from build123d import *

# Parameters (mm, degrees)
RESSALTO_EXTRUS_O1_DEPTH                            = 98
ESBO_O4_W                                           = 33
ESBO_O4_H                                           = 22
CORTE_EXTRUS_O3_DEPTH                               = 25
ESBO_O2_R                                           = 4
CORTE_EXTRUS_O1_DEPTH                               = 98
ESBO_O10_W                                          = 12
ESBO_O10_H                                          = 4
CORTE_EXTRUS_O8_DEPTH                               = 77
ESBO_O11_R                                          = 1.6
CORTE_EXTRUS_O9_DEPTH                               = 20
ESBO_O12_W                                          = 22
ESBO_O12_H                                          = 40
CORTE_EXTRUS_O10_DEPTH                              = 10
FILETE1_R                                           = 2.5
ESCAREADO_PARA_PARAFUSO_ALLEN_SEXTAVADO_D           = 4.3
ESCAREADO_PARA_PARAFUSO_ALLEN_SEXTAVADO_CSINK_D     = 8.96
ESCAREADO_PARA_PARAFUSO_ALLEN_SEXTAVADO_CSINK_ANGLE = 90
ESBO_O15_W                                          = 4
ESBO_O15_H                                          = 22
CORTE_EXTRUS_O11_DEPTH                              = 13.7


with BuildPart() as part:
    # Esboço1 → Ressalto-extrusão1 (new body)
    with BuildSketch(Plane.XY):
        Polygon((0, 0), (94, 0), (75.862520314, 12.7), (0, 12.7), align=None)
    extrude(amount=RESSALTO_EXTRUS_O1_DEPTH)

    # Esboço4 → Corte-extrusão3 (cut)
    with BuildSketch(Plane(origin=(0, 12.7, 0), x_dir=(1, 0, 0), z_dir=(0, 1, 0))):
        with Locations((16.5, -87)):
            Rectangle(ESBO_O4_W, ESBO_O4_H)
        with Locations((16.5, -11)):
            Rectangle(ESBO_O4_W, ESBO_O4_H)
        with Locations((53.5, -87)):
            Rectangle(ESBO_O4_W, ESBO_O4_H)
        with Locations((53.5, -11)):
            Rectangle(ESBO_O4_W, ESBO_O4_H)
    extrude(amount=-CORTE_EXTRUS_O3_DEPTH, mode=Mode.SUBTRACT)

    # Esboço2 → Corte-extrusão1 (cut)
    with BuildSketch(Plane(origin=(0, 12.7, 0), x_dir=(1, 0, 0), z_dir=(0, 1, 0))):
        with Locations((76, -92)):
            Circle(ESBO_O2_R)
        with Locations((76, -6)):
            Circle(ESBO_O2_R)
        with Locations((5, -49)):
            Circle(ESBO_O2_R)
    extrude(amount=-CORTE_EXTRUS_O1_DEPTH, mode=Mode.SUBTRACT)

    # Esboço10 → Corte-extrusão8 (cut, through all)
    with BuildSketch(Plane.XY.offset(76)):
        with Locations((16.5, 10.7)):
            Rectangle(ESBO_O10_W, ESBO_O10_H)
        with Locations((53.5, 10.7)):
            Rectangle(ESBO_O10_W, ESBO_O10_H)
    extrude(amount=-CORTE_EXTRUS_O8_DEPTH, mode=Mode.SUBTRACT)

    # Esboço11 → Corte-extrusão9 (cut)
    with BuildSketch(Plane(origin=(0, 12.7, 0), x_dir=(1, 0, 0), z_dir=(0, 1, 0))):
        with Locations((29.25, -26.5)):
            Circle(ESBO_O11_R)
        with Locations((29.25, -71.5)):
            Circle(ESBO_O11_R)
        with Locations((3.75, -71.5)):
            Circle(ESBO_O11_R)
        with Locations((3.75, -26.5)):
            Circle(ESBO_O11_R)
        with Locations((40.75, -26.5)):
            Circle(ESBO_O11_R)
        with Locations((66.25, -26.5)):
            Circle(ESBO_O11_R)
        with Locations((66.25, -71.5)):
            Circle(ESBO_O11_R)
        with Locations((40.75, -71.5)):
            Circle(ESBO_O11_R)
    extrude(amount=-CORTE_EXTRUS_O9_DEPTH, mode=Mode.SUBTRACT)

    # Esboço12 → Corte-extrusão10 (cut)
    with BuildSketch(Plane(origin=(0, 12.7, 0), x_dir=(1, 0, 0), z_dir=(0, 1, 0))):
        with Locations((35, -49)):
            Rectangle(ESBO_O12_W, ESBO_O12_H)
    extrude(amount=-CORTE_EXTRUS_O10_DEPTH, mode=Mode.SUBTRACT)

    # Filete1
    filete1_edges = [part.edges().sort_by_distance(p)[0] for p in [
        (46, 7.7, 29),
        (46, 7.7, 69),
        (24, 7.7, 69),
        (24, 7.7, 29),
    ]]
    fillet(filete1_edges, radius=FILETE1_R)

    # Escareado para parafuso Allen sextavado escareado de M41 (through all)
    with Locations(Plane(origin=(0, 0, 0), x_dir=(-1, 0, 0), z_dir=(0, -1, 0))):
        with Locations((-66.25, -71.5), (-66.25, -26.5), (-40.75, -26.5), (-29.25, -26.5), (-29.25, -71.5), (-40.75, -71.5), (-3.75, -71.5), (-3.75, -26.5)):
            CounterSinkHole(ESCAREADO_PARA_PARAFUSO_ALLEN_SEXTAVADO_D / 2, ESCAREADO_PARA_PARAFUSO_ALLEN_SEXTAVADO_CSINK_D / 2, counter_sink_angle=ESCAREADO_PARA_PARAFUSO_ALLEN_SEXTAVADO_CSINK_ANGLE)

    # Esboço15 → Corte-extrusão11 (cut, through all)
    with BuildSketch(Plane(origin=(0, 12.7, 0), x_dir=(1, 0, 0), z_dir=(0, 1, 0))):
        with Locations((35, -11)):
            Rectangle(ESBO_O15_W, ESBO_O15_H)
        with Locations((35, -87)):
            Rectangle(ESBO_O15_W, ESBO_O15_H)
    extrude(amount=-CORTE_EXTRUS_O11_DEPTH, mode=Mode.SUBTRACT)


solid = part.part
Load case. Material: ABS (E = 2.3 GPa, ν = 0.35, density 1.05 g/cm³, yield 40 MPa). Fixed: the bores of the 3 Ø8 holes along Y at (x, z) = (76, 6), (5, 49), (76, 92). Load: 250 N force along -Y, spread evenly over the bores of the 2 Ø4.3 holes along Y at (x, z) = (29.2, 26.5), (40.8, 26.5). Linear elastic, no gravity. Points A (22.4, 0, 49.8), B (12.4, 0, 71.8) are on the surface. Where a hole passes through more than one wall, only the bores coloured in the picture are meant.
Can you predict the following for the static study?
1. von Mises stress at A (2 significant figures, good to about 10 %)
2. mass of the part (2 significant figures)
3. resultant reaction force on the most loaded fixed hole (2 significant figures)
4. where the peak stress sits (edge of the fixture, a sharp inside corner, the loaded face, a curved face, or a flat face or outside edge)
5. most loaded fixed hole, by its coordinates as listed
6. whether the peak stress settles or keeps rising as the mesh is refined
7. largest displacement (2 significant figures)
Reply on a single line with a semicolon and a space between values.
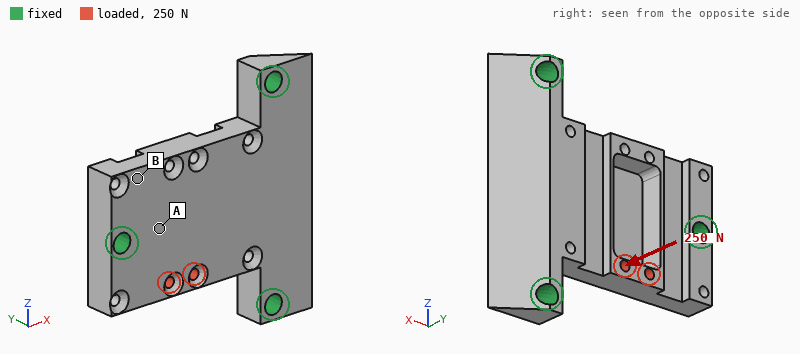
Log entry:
2.8 MPa; 51 g; 170 N; a sharp inside corner; (5, 49); keeps rising; 0.32 mm
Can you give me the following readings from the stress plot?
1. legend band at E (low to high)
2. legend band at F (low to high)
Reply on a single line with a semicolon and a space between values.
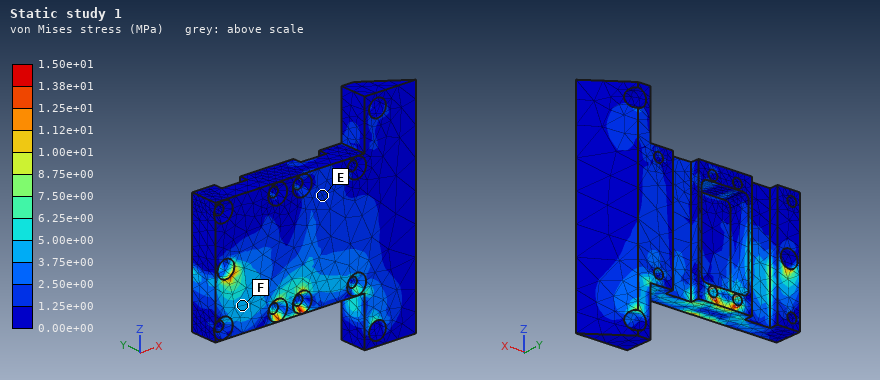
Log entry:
1.25e+00 to 2.50e+00 MPa; 3.75e+00 to 5.00e+00 MPa
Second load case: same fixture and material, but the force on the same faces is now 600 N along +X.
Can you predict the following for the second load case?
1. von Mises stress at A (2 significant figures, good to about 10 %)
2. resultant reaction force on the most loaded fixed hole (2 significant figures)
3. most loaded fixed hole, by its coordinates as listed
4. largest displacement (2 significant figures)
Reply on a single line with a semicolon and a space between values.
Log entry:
2.1 MPa; 430 N; (5, 49); 0.14 mm
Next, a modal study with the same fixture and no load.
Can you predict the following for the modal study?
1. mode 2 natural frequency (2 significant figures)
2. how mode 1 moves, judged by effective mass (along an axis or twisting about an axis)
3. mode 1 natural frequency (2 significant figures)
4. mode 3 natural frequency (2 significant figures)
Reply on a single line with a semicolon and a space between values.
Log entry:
2500 Hz; along Y; 1500 Hz; 2500 Hz
